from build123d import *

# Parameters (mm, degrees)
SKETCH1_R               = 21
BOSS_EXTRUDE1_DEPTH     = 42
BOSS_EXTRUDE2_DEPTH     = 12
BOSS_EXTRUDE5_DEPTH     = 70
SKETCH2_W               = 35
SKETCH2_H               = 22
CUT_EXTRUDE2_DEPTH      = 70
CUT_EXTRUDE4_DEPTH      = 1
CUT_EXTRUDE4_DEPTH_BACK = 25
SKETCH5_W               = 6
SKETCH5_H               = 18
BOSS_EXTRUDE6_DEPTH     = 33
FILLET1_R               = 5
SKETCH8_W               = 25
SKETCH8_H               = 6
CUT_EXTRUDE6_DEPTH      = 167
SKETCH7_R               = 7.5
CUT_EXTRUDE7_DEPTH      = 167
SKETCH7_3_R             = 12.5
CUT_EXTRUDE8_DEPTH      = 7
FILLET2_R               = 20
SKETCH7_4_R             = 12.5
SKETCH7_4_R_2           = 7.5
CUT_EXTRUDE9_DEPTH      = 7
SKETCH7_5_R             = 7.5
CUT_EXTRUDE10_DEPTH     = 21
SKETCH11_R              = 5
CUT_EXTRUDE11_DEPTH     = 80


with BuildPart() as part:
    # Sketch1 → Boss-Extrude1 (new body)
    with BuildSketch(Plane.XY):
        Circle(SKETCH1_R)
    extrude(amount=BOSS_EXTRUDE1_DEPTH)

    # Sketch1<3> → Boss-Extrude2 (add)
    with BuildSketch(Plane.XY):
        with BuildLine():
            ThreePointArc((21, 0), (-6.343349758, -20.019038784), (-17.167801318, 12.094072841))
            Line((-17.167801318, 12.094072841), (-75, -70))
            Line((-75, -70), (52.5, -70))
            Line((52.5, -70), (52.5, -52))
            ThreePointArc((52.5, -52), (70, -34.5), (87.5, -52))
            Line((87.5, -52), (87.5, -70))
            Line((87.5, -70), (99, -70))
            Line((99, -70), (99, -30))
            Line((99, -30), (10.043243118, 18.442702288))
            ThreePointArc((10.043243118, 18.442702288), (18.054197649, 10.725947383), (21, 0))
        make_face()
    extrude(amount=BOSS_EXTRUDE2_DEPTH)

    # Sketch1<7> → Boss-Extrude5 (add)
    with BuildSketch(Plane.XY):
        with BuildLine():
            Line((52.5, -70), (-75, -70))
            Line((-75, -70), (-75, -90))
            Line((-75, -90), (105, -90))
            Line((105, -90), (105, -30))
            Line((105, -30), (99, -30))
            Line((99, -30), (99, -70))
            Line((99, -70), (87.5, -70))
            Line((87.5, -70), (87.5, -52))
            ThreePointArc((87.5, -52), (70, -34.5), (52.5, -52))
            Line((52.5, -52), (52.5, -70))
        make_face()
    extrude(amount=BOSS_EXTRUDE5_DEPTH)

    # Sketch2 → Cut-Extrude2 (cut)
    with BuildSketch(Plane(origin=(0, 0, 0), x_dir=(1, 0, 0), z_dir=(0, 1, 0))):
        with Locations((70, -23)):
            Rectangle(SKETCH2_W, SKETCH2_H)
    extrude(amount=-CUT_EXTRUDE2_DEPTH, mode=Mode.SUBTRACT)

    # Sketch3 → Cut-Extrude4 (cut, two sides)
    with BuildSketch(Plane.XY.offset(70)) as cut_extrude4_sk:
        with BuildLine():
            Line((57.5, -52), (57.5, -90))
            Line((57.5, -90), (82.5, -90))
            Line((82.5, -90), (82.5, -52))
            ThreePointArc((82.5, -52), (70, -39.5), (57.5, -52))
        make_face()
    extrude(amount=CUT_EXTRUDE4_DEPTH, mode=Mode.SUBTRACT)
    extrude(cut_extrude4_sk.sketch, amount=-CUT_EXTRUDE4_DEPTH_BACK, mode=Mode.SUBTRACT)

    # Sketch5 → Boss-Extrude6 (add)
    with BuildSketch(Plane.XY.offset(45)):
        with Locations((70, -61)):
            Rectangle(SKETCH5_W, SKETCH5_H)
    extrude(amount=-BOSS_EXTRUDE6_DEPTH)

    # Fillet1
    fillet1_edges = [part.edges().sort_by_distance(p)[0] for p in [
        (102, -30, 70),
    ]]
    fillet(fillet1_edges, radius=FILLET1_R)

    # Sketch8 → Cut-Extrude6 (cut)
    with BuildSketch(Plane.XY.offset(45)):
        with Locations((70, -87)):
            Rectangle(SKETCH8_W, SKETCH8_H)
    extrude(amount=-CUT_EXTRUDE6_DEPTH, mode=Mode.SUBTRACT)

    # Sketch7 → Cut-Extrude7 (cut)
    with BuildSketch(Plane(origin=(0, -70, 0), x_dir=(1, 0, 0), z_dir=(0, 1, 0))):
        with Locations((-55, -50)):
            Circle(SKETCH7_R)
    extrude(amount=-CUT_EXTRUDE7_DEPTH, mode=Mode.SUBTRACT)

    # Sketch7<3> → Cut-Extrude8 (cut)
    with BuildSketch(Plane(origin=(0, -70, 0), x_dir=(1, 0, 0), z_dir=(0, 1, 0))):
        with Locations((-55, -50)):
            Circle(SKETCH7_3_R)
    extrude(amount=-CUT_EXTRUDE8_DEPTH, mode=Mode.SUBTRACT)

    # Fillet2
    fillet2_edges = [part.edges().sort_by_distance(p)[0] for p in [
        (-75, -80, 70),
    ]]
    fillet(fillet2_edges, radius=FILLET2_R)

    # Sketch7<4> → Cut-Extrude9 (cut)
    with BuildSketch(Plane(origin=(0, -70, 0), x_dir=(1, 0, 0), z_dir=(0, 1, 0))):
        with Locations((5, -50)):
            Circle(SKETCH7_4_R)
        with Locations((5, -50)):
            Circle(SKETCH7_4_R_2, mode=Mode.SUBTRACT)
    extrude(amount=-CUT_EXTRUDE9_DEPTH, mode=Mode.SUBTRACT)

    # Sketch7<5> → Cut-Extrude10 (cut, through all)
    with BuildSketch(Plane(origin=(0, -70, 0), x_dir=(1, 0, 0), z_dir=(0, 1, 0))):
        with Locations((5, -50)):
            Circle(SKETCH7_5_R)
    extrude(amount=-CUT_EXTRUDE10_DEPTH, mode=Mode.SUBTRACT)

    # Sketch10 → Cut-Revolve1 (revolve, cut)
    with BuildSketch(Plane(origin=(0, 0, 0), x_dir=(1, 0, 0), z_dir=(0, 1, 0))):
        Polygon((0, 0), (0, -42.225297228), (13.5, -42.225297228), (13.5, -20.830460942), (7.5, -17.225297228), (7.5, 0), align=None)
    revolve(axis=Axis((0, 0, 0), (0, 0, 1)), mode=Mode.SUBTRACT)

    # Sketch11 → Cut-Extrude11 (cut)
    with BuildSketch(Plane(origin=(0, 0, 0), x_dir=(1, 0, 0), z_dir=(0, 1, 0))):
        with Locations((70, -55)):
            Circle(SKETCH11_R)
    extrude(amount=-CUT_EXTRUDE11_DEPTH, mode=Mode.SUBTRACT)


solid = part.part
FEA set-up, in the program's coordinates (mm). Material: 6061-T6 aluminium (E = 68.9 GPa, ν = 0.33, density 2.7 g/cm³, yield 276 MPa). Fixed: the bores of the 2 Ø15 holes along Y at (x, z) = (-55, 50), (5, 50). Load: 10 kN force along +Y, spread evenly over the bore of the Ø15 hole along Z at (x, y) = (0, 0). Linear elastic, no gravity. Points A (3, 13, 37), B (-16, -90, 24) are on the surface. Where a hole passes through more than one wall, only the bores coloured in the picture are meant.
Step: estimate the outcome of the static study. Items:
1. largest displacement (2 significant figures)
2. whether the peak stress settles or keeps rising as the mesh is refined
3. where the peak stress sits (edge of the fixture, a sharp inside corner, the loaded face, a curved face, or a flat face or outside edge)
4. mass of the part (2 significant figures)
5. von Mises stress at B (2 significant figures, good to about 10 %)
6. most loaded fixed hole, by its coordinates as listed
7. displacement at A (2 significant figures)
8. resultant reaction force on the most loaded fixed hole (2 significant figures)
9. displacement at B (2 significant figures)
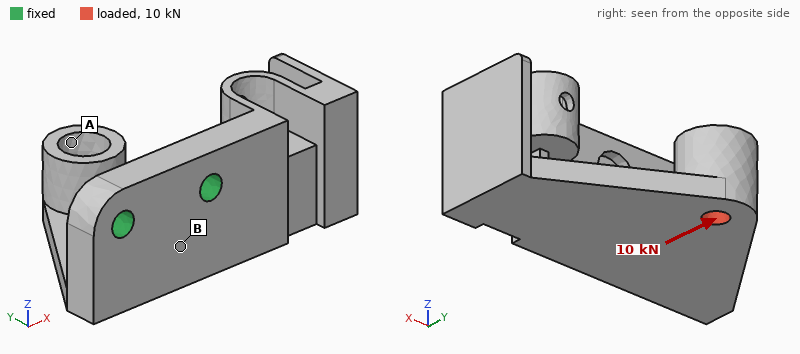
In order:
0.25 mm
keeps rising
edge of the fixture
1.1 kg
25 MPa
(5, 50)
0.22 mm
8.2 kN
0.054 mm
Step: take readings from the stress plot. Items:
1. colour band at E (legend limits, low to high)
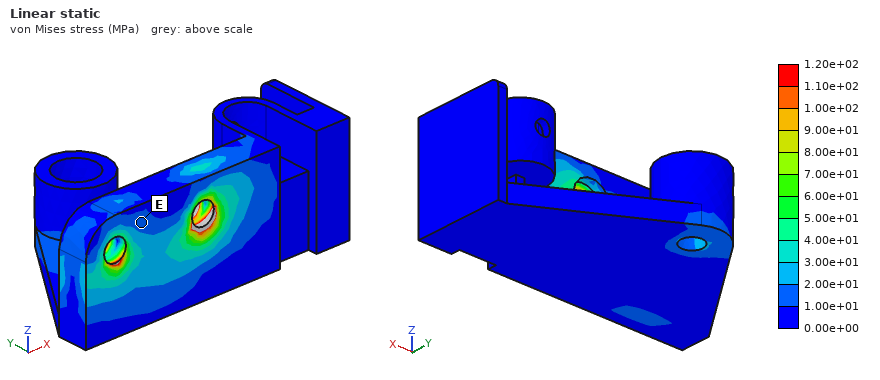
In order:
1.00e+01 to 2.00e+01 MPa
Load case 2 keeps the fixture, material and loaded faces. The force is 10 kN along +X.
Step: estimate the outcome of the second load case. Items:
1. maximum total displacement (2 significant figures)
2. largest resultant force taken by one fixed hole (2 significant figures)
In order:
0.46 mm
14 kN
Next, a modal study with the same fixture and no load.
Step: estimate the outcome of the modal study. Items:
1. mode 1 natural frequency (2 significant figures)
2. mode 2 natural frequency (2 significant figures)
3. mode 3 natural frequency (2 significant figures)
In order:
860 Hz
1200 Hz
1900 Hz
